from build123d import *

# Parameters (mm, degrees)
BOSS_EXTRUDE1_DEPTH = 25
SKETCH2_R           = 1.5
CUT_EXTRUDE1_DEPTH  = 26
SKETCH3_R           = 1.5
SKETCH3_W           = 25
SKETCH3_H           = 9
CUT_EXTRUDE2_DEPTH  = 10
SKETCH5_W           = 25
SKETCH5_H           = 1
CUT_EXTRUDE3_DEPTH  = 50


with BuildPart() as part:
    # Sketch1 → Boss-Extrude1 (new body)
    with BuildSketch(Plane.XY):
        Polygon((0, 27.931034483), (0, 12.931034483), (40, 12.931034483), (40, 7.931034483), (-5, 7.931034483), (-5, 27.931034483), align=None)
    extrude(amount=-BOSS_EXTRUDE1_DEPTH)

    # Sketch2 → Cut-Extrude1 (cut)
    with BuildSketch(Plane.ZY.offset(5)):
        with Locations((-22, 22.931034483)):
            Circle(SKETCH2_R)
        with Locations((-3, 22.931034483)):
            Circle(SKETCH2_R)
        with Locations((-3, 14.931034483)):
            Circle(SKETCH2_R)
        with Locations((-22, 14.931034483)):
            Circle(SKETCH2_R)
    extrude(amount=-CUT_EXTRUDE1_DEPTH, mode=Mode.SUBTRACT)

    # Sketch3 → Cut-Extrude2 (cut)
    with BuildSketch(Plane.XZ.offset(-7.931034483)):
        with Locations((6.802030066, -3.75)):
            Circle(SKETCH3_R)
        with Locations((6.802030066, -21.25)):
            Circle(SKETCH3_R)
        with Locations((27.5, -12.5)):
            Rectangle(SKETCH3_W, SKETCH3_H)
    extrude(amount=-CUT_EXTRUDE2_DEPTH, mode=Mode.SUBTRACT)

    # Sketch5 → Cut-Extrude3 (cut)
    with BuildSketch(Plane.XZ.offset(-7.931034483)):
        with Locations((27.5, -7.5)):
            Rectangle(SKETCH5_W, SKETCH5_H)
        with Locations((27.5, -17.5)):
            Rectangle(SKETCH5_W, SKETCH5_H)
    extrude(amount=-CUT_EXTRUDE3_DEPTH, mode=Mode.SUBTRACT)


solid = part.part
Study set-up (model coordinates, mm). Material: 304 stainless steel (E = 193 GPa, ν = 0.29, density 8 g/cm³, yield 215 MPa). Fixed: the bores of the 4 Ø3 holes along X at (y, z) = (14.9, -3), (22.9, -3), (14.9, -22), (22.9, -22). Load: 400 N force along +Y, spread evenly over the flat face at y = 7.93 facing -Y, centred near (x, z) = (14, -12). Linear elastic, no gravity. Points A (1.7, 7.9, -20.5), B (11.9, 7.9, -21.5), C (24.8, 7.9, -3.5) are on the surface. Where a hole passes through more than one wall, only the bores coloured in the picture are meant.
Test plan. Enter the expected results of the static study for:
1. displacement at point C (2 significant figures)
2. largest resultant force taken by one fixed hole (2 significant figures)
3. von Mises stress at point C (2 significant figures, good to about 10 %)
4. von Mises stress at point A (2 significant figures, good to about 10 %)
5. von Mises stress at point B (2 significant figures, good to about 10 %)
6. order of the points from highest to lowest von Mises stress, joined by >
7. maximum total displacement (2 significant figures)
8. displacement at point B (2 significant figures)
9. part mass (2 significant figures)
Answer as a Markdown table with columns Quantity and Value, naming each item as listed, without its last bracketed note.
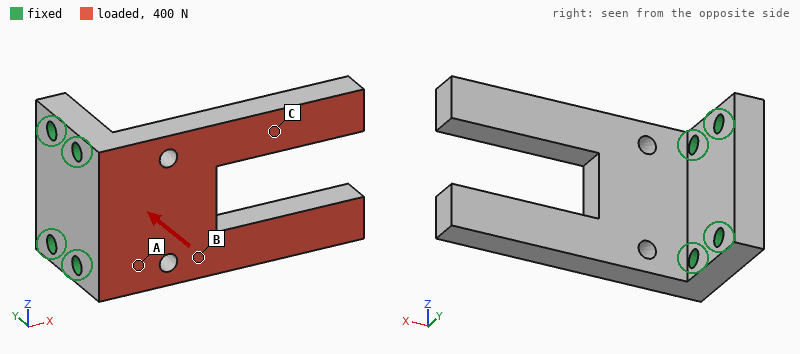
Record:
| Quantity | Value |
|---|---|
| displacement at point C | 47 µm |
| largest resultant force taken by one fixed hole | 190 N |
| von Mises stress at point C | 14 MPa |
| von Mises stress at point A | 48 MPa |
| von Mises stress at point B | 31 MPa |
| order of the points from highest to lowest von Mises stress, joined by > | A > B > C |
| maximum total displacement | 88 µm |
| displacement at point B | 18 µm |
| part mass | 47 g |
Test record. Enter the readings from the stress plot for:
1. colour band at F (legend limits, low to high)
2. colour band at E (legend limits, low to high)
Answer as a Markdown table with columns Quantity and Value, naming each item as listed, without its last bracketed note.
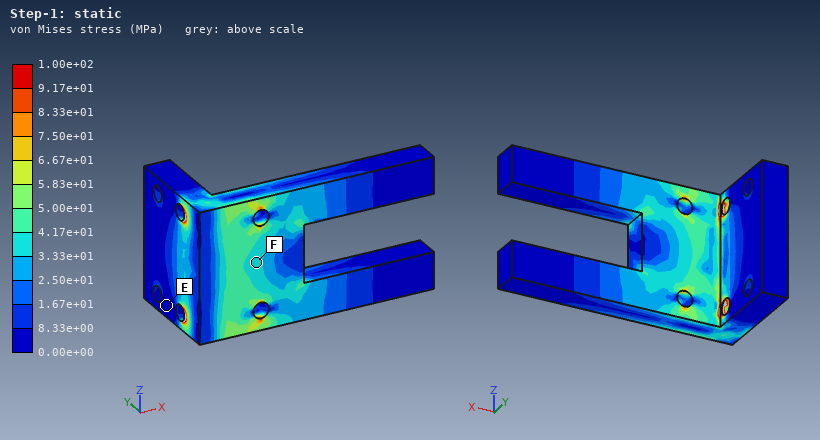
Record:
| Quantity | Value |
|---|---|
| colour band at F | 3.33e+01 to 4.17e+01 MPa |
| colour band at E | 0.00e+00 to 8.33e+00 MPa |
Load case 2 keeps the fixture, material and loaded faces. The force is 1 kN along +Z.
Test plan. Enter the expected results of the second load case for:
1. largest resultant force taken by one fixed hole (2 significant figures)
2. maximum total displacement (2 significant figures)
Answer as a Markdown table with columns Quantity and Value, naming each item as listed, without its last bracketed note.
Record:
| Quantity | Value |
|---|---|
| largest resultant force taken by one fixed hole | 1.0 kN |
| maximum total displacement | 41 µm |
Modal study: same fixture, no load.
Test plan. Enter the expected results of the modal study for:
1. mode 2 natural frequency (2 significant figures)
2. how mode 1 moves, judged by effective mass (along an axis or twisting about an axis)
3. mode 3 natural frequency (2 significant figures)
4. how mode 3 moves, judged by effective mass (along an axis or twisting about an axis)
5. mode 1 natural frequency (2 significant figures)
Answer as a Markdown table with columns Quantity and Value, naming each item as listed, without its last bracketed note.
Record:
| Quantity | Value |
|---|---|
| mode 2 natural frequency | 3500 Hz |
| how mode 1 moves, judged by effective mass | along Y |
| mode 3 natural frequency | 5500 Hz |
| how mode 3 moves, judged by effective mass | along Z |
| mode 1 natural frequency | 2400 Hz |
